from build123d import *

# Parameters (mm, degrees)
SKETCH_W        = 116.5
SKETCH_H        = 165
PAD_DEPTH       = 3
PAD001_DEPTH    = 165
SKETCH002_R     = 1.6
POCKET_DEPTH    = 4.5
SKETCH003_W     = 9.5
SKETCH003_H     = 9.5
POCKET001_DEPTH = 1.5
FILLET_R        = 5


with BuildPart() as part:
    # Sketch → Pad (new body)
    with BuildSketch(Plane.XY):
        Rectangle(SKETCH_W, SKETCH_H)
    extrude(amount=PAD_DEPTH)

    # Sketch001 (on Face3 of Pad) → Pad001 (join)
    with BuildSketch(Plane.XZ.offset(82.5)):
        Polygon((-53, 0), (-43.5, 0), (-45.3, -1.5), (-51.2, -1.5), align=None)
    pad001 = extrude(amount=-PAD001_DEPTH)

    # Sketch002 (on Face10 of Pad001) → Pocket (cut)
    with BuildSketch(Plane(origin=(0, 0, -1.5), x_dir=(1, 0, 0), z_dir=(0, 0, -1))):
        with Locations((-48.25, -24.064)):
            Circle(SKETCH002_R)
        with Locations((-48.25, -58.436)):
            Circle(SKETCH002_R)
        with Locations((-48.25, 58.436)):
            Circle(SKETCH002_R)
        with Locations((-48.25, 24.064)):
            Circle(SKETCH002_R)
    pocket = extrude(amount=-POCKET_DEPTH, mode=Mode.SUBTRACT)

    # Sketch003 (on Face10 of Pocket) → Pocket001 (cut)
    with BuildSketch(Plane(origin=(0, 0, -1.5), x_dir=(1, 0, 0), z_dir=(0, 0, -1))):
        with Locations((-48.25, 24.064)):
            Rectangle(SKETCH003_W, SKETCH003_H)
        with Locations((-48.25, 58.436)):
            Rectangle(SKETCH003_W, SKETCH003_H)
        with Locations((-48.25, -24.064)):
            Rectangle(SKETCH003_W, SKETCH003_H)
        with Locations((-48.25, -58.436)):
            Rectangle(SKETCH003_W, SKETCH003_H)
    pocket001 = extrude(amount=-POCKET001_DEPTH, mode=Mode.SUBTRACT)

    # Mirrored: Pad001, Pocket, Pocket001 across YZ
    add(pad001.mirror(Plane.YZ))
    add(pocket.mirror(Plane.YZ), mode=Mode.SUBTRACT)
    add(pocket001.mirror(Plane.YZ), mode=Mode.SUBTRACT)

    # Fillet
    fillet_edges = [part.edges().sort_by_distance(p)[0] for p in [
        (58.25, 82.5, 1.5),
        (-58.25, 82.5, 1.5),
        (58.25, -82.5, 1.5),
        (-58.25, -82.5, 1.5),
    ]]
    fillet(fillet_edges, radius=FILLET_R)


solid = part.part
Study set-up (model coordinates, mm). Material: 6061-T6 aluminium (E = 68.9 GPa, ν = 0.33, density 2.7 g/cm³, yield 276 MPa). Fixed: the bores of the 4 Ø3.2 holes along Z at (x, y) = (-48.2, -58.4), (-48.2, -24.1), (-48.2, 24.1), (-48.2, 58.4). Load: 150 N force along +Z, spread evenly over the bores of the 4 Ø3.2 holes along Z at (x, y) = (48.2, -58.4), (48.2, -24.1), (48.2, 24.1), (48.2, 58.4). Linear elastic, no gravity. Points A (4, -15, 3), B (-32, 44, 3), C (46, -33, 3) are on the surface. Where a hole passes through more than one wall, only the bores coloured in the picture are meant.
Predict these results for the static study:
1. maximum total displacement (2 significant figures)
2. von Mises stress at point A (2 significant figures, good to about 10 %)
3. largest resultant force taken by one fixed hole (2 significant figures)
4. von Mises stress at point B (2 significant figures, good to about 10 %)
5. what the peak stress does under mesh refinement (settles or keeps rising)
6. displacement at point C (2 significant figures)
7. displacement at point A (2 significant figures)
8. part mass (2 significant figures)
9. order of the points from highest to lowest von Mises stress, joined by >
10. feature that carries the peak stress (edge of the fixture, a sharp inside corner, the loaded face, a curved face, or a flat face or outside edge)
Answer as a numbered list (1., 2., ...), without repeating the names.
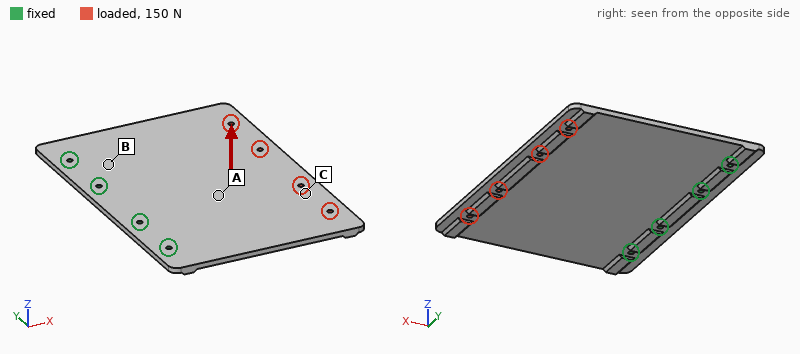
1. 2.1 mm
2. 24 MPa
3. 57 N
4. 46 MPa
5. keeps rising
6. 1.7 mm
7. 0.68 mm
8. 160 g
9. B > A > C
10. edge of the fixture
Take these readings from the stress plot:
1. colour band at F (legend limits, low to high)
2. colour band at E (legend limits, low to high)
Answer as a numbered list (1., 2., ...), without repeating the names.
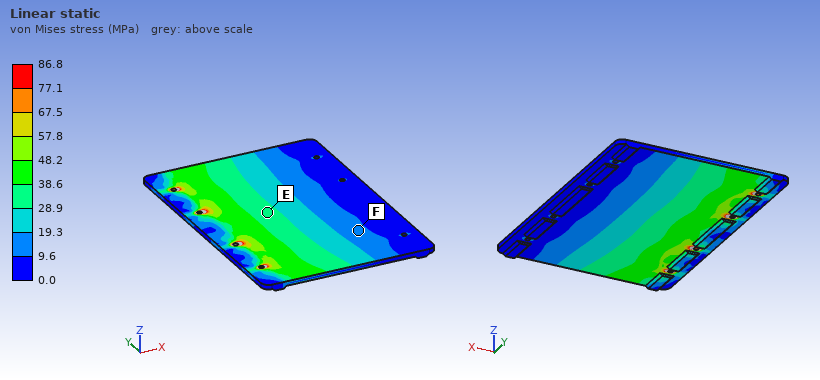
1. 9.6 to 19.3 MPa
2. 28.9 to 38.6 MPa
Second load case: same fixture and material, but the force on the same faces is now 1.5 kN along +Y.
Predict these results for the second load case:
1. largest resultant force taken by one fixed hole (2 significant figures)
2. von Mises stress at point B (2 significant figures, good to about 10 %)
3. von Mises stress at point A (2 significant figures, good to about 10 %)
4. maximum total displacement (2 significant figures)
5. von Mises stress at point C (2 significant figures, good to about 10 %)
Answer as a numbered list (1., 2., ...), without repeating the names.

1. 1.1 kN
2. 9.9 MPa
3. 8.5 MPa
4. 34 µm
5. 4.9 MPa
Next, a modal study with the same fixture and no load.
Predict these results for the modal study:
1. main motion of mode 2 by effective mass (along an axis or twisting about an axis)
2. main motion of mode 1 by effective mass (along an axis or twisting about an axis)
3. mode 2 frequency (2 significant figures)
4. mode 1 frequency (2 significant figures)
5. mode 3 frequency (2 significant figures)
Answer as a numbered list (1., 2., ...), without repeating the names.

1. twisting about X
2. along Z
3. 380 Hz
4. 210 Hz
5. 880 Hz
